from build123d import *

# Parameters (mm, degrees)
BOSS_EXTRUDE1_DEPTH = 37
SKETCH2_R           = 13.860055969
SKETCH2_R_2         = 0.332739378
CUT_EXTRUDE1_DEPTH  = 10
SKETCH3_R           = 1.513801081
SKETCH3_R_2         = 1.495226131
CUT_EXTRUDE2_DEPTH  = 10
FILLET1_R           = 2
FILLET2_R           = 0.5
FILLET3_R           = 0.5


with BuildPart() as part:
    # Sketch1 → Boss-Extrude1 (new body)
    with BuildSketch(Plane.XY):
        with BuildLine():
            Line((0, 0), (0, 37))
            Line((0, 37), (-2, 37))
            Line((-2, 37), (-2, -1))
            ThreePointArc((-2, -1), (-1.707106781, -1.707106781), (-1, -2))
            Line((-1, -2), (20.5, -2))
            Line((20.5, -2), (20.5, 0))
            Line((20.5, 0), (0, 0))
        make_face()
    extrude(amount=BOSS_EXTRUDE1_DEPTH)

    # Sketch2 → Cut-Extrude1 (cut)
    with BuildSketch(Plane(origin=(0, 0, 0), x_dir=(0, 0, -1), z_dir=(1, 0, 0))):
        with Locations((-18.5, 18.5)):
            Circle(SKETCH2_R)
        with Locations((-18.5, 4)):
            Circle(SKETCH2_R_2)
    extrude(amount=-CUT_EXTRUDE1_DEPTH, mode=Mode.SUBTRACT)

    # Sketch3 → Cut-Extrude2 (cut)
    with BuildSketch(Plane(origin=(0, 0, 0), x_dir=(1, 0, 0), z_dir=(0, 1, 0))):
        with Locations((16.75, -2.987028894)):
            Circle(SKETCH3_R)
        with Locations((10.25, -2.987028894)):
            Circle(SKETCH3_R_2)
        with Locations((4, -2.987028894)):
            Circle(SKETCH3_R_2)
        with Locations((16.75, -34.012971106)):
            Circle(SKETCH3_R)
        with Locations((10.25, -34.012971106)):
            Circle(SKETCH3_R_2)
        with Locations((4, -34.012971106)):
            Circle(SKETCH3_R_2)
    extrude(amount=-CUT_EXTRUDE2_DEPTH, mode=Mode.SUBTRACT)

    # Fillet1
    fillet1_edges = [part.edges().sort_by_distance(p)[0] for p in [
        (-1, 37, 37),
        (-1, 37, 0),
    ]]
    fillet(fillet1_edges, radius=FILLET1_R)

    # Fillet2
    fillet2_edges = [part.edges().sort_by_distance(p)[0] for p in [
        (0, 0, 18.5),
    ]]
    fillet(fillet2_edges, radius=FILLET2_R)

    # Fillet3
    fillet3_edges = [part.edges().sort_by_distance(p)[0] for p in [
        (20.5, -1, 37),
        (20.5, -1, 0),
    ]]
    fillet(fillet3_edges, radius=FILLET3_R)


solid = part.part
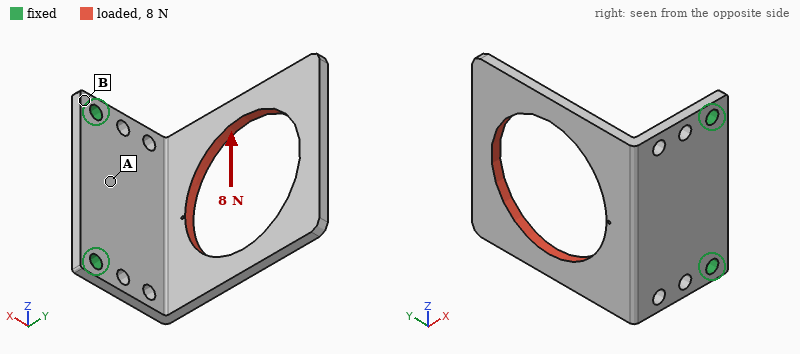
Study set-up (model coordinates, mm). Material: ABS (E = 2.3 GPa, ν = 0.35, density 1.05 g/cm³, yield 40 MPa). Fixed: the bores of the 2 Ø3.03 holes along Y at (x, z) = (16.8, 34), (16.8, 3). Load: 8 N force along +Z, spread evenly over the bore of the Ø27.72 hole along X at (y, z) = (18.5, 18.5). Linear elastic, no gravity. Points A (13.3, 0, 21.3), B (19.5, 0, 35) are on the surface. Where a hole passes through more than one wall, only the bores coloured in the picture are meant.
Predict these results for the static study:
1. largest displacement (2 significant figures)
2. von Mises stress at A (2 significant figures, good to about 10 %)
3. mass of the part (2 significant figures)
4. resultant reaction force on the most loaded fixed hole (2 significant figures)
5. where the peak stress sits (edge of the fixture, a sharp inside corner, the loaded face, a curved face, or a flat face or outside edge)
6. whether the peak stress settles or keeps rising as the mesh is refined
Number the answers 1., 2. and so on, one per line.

1. 0.63 mm
2. 1.6 MPa
3. 3.3 g
4. 8.0 N
5. edge of the fixture
6. keeps rising
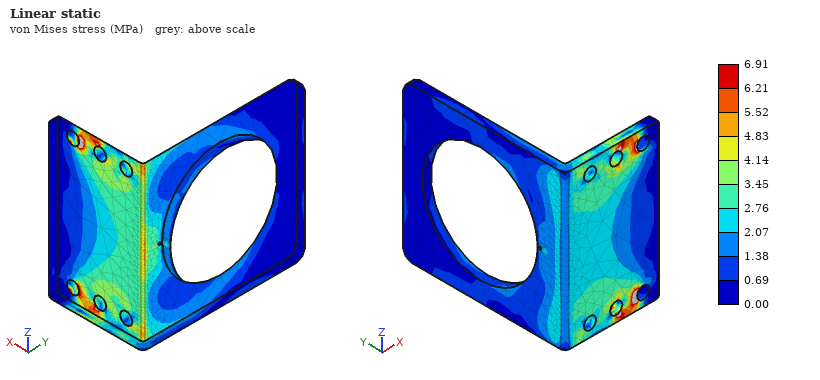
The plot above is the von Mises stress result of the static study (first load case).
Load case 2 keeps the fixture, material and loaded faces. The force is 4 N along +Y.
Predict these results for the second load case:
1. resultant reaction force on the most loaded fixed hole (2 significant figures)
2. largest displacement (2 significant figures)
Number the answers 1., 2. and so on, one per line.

1. 2.0 N
2. 0.60 mm
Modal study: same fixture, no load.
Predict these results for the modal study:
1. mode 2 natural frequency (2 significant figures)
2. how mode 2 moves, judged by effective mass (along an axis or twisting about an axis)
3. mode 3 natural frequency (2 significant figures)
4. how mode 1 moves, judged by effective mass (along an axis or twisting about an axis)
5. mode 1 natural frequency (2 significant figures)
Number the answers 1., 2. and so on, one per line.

1. 450 Hz
2. along Z
3. 640 Hz
4. along X
5. 190 Hz
